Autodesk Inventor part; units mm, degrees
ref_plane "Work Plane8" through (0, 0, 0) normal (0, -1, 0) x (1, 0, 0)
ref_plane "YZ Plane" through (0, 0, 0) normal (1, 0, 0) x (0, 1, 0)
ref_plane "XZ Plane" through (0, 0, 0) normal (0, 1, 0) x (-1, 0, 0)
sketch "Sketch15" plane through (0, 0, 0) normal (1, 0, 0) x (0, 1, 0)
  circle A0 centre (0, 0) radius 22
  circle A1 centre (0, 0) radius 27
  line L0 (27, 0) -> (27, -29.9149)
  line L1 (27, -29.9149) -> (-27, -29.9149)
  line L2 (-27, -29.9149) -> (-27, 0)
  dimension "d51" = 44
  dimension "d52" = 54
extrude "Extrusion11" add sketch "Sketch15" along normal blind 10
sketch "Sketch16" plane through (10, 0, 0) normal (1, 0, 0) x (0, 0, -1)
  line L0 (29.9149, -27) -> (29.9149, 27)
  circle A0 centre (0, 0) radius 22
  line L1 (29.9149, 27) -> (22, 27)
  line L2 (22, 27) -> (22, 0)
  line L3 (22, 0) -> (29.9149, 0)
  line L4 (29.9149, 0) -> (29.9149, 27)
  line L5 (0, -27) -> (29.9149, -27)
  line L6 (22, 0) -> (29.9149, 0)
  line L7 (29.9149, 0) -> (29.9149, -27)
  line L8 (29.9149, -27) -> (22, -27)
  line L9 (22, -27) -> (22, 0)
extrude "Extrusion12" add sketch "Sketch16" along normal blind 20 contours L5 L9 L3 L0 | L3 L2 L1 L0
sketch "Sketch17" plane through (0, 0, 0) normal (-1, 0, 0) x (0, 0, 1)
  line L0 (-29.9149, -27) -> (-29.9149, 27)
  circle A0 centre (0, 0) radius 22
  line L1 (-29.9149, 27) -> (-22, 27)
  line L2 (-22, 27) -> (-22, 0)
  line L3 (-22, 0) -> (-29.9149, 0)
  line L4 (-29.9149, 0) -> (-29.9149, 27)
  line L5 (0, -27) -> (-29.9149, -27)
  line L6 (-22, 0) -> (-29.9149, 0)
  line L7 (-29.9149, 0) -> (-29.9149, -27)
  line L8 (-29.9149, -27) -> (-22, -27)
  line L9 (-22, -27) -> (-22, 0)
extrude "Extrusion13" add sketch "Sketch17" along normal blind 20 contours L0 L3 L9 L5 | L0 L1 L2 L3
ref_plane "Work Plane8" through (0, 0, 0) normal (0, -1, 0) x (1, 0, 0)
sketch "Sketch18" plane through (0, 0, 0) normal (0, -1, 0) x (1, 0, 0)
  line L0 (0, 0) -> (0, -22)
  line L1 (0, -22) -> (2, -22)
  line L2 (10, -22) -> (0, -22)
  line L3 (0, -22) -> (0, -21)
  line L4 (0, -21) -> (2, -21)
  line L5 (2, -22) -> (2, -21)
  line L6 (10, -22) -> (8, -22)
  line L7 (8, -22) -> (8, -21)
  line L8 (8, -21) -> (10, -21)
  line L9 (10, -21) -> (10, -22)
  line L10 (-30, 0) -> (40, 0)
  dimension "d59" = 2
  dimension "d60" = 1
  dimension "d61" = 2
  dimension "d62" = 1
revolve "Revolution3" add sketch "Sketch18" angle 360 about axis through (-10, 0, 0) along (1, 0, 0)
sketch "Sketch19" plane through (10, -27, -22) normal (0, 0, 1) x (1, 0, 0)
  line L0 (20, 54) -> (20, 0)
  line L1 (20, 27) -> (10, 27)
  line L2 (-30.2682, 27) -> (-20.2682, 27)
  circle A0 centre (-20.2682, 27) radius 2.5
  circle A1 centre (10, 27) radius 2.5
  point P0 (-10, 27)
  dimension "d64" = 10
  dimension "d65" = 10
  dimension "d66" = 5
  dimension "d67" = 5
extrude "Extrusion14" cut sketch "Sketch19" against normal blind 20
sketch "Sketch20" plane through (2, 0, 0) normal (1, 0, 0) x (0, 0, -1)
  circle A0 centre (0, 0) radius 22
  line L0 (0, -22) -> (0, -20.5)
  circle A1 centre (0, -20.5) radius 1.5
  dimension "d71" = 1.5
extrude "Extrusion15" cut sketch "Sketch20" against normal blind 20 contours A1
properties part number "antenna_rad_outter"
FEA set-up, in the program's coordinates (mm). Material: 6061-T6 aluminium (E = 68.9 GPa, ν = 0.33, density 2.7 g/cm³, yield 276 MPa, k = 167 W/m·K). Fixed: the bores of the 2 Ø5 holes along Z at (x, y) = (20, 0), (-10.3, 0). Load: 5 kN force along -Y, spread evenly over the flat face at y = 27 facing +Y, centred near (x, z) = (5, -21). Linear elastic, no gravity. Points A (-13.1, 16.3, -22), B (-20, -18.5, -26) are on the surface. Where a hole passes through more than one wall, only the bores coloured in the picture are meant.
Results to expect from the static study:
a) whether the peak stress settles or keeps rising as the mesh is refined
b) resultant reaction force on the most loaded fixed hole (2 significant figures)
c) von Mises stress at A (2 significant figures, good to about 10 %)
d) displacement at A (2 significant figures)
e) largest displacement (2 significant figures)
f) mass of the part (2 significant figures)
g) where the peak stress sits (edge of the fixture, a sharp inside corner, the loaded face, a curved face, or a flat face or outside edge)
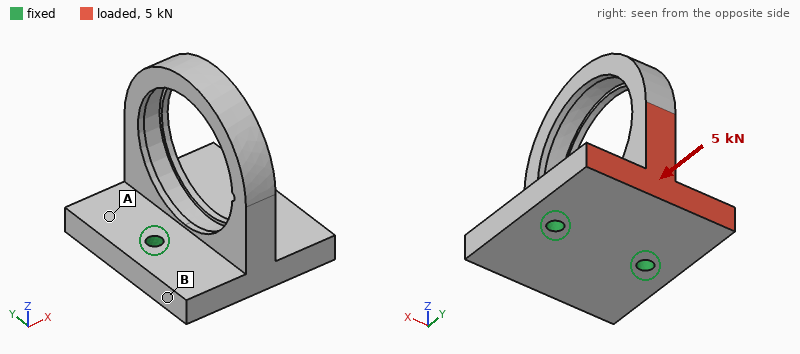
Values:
keeps rising
2.5 kN
27 MPa
0.023 mm
0.12 mm
80 g
edge of the fixture
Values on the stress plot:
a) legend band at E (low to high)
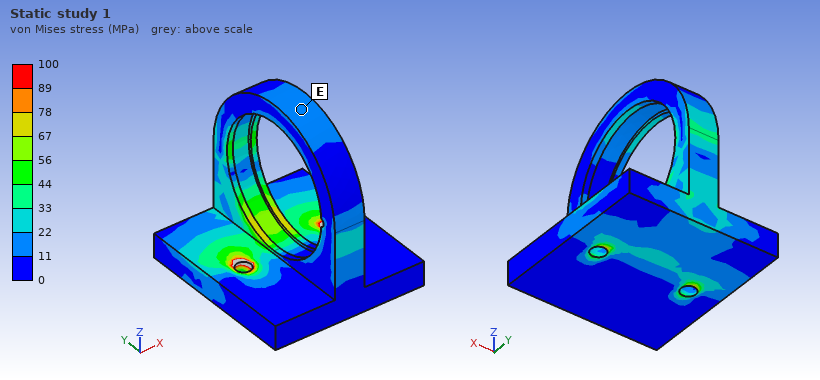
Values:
11 to 22 MPa
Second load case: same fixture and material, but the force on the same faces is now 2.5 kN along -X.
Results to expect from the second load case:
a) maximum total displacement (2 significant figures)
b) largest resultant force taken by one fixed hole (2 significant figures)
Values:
73 µm
2.4 kN
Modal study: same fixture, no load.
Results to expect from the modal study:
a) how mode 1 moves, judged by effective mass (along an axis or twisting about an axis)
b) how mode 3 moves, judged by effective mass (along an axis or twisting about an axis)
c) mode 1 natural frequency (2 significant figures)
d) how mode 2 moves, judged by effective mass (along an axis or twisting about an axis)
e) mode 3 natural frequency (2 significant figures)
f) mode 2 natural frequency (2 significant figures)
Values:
along X
along Z
2600 Hz
along Y
5600 Hz
2900 Hz
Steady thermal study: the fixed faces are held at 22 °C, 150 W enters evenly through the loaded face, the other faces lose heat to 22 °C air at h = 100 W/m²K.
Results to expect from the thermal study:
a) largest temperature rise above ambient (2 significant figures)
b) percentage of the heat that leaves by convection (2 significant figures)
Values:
68 K
15 %
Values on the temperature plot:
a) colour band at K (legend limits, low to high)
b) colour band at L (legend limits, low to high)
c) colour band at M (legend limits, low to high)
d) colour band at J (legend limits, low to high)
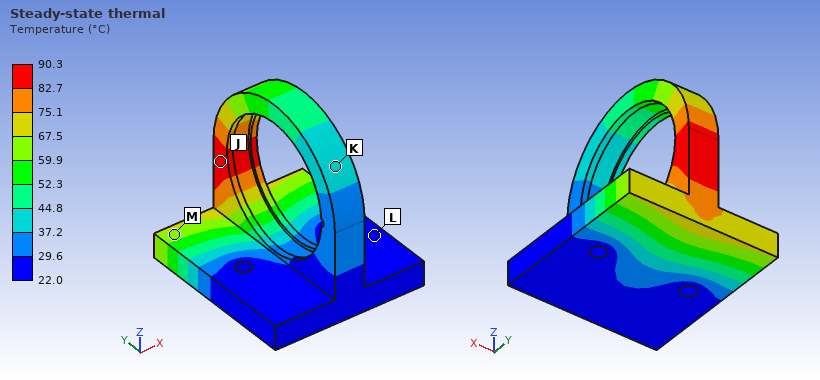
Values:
37.2 to 44.8 °C
22.0 to 29.6 °C
59.9 to 67.5 °C
82.7 to 90.3 °C
